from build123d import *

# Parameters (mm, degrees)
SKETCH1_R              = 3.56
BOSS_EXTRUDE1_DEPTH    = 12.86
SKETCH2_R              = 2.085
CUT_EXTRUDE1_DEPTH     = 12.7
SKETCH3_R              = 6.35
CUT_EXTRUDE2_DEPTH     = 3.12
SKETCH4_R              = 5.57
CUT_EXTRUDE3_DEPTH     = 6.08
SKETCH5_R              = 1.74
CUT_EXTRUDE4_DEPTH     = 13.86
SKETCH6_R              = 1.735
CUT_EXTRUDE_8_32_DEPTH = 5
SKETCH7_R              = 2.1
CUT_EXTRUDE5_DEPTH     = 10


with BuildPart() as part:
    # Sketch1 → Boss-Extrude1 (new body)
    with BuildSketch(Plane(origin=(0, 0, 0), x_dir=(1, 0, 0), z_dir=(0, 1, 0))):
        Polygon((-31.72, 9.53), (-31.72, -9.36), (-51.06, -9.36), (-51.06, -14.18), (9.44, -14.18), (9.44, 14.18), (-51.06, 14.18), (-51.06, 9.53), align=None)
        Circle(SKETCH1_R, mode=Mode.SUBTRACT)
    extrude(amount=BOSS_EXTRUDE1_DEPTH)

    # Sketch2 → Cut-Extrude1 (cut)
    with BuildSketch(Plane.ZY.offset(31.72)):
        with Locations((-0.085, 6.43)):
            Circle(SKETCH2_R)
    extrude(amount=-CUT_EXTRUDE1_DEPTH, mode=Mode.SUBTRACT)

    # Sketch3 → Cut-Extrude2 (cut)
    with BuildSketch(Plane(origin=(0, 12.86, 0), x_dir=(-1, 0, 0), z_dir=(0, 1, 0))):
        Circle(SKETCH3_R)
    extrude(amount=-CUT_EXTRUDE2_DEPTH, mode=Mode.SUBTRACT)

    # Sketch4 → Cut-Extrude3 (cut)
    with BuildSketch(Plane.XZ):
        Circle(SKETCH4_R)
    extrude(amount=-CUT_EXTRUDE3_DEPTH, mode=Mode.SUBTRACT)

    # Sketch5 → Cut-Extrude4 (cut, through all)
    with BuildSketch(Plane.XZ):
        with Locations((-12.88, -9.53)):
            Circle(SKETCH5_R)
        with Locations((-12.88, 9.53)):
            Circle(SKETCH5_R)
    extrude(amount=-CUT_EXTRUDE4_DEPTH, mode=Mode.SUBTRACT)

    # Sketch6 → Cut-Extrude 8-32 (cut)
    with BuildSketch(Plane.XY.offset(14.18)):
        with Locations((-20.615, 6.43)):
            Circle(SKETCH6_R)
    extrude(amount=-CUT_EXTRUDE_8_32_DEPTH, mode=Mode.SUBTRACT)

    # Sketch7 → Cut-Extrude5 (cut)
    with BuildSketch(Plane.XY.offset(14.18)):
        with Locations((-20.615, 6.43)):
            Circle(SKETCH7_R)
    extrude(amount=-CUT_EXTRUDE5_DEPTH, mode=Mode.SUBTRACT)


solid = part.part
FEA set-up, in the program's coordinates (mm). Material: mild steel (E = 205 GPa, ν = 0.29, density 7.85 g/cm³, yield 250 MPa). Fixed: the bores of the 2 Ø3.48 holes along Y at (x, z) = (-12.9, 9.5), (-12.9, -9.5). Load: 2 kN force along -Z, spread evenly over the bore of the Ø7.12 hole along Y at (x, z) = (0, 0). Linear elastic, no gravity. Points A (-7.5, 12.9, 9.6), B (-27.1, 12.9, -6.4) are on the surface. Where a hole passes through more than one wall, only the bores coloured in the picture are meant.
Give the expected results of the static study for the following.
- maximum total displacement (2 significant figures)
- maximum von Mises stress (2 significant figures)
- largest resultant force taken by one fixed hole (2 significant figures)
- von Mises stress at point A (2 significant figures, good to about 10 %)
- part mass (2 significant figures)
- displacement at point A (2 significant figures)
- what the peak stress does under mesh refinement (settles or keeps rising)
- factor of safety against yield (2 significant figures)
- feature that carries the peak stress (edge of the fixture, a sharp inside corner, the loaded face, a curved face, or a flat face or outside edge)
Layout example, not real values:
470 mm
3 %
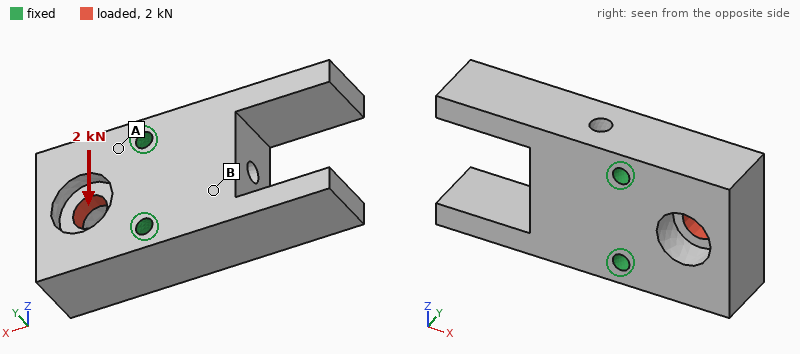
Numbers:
3.3 µm
54 MPa
1.5 kN
10 MPa
120 g
0.59 µm
settles
4.7
the loaded face
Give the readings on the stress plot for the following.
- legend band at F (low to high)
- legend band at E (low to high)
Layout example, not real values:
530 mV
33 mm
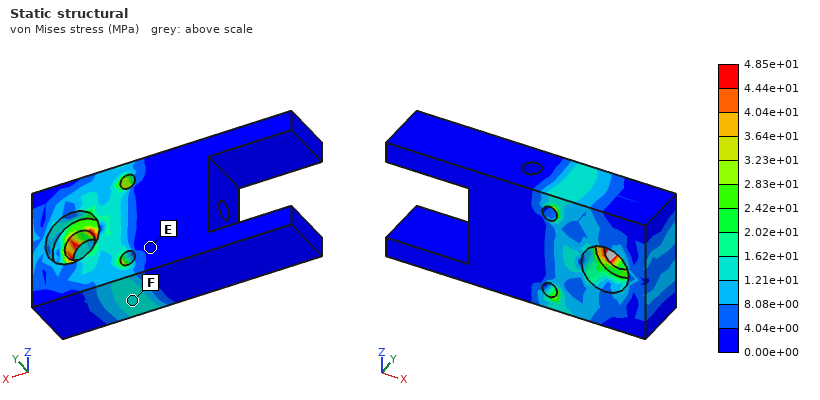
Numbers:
1.21e+01 to 1.62e+01 MPa
0.00e+00 to 4.04e+00 MPa
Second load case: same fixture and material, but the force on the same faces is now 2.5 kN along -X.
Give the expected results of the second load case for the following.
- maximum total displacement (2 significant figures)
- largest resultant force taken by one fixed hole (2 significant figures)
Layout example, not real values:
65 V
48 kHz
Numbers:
2.2 µm
1.3 kN
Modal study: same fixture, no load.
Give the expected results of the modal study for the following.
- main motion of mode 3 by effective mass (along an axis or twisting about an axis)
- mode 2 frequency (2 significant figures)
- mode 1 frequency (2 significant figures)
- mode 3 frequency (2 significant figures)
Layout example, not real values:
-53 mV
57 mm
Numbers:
along Y
7800 Hz
7500 Hz
9200 Hz
